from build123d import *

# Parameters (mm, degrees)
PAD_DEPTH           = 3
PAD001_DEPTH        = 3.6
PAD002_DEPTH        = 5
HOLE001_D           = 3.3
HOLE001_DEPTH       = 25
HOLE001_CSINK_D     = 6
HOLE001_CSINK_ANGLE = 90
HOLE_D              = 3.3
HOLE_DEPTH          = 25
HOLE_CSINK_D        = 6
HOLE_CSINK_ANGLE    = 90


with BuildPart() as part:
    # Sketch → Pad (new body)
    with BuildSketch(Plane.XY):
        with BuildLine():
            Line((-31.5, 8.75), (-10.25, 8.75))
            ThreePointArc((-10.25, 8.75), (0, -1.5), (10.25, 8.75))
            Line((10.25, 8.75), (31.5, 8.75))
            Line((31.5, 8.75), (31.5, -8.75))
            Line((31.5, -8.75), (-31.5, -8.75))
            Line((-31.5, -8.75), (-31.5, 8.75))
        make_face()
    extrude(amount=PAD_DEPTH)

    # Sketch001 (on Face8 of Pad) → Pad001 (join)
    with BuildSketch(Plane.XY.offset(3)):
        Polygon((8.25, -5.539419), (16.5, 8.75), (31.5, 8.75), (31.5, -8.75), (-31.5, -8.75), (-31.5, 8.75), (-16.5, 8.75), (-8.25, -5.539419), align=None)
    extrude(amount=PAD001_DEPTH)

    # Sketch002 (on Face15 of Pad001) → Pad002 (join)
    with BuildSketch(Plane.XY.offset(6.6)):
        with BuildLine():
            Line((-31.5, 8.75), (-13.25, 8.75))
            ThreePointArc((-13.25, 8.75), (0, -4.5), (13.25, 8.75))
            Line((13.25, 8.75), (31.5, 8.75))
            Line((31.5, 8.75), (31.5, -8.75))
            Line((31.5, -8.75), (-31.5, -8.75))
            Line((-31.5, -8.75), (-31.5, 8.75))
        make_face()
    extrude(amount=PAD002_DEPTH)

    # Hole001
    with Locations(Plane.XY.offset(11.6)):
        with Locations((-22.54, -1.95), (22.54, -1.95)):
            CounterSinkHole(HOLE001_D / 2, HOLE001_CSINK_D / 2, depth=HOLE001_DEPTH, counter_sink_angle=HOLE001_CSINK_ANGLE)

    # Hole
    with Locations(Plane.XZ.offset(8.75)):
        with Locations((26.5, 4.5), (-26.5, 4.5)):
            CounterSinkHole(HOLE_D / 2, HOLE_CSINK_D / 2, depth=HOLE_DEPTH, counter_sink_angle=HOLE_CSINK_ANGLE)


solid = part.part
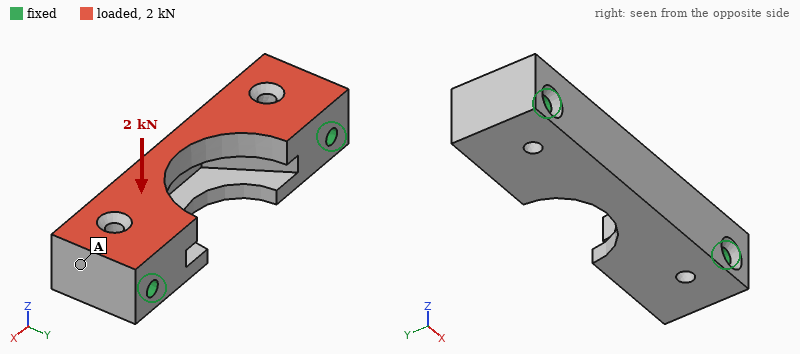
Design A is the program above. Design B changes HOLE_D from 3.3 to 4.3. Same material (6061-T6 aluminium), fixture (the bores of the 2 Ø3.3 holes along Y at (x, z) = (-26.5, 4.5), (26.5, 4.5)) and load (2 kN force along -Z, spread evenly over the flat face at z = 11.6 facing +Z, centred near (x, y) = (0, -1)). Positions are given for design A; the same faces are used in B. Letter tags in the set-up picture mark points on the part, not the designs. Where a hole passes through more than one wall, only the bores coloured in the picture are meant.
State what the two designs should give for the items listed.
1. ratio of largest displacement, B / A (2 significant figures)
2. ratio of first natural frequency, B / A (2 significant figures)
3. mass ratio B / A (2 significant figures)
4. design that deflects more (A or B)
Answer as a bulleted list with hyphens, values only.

- 0.81
- 1.1
- 0.98
- A
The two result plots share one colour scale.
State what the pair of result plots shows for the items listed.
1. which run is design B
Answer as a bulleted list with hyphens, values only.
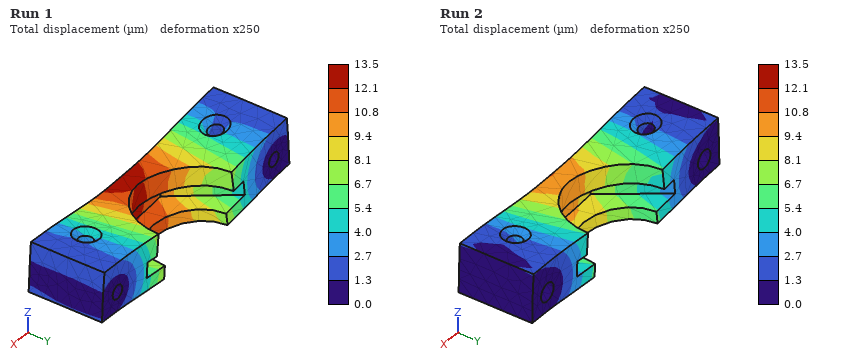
- Run 2
